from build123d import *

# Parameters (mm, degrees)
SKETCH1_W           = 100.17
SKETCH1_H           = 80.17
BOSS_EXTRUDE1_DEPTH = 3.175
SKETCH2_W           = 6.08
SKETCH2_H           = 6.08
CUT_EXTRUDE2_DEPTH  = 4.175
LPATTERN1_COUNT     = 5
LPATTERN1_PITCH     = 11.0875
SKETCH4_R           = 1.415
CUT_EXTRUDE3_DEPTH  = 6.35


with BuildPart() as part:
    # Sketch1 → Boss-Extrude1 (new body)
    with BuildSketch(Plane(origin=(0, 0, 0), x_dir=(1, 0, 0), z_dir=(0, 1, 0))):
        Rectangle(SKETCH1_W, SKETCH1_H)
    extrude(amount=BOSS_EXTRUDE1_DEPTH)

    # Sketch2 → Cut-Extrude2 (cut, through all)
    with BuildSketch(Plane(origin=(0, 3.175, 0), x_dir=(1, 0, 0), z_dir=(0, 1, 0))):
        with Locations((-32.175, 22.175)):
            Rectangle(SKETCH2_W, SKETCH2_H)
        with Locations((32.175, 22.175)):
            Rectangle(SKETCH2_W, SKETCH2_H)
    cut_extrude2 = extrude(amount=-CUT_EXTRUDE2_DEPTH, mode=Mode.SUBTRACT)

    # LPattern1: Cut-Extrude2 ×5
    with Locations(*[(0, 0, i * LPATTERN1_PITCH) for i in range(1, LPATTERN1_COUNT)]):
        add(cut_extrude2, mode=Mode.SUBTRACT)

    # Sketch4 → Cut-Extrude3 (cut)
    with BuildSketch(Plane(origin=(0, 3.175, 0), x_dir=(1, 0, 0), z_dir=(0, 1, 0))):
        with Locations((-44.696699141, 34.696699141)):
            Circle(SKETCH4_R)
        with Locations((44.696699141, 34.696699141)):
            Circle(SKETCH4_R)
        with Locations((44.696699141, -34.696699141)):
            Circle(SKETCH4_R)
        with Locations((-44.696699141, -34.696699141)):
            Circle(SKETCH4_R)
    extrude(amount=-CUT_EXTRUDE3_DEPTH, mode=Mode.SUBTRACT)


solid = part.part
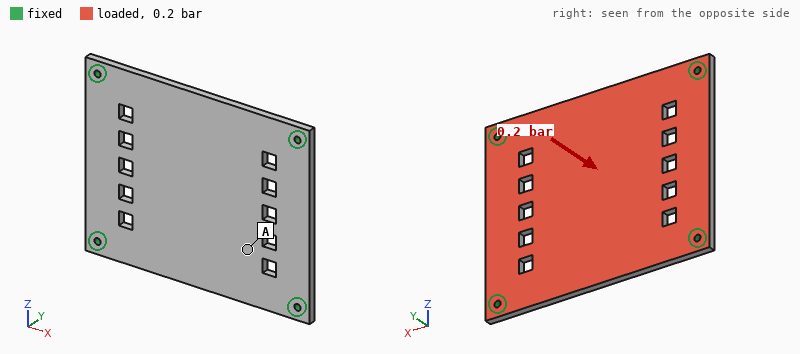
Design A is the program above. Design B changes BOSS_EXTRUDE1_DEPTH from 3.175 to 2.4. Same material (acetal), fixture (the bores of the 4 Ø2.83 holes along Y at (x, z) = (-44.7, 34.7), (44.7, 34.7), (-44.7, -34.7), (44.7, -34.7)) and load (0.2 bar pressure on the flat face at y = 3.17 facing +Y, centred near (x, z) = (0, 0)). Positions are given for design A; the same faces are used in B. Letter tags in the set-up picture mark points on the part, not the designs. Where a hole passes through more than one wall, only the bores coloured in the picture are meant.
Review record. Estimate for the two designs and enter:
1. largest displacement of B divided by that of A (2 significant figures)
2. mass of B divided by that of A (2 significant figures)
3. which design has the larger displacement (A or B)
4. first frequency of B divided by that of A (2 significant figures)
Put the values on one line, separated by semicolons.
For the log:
2.2; 0.76; B; 0.77
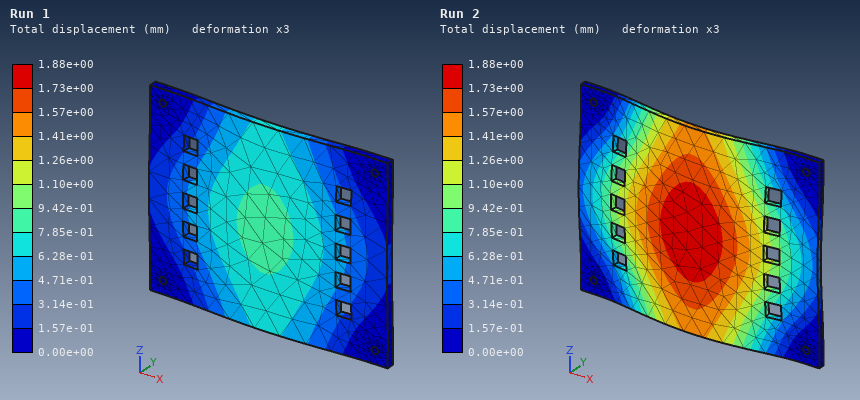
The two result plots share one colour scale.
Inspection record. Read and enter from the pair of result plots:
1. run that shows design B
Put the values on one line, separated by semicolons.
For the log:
Run 2
